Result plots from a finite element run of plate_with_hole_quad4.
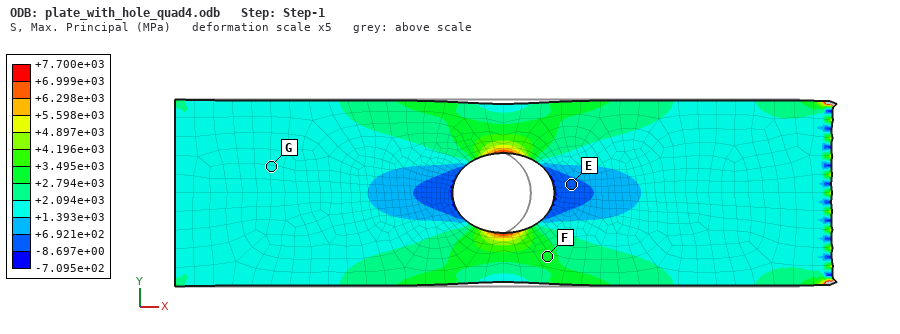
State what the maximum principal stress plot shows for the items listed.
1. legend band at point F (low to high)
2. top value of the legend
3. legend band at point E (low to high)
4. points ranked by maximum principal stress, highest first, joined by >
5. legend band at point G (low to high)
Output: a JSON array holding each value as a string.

["+2.794e+03 to +3.495e+03 MPa", "+7.700e+03 MPa", "-8.697e+00 to +6.921e+02 MPa", "F > G > E", "+1.393e+03 to +2.094e+03 MPa"]
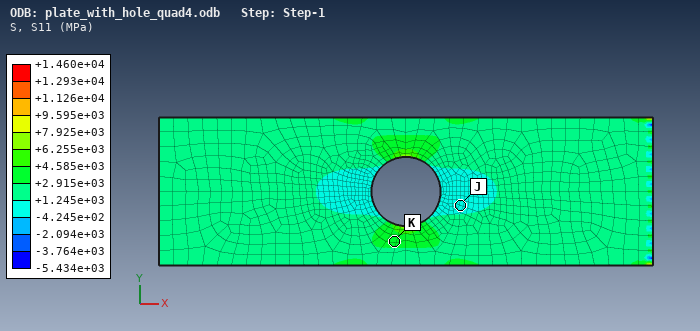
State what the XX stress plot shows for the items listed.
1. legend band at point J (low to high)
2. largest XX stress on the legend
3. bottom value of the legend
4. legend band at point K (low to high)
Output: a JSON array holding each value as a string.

["-4.245e+02 to +1.245e+03 MPa", "+1.460e+04 MPa", "-5.434e+03 MPa", "+2.915e+03 to +4.585e+03 MPa"]
